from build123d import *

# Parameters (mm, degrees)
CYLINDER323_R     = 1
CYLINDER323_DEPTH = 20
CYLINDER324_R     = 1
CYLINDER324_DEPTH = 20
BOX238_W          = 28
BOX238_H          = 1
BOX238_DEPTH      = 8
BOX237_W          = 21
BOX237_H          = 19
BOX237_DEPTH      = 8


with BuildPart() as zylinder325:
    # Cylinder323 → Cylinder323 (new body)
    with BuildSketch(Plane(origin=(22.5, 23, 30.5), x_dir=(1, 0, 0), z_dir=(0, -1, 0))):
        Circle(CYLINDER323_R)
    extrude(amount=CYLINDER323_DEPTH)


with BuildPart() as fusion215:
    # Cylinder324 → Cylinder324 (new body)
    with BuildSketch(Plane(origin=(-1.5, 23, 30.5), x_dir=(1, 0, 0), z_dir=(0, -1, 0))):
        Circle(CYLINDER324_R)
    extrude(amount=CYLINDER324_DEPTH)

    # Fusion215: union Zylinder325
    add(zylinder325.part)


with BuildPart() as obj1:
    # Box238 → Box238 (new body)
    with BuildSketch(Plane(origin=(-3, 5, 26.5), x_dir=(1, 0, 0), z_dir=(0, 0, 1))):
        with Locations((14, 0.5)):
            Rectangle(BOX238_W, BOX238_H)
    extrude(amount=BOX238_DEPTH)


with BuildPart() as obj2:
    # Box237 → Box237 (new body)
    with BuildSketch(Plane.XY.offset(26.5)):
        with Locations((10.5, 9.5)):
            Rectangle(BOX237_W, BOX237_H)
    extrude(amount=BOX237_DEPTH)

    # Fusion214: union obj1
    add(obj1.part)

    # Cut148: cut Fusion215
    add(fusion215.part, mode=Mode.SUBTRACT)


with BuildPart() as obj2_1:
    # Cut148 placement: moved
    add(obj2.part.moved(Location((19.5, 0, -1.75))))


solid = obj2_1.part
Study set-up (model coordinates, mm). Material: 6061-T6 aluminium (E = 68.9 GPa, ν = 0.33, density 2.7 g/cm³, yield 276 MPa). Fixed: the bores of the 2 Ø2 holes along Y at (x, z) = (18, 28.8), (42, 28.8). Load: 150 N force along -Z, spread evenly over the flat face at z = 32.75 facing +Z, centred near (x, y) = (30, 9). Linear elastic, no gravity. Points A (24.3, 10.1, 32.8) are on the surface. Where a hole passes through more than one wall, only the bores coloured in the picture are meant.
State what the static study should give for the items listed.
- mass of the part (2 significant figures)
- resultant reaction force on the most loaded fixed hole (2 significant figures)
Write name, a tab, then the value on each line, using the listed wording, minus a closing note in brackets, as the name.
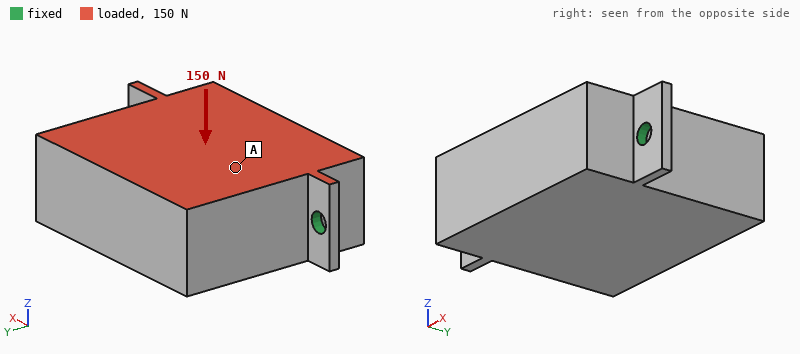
mass of the part	8.8 g
resultant reaction force on the most loaded fixed hole	75 N
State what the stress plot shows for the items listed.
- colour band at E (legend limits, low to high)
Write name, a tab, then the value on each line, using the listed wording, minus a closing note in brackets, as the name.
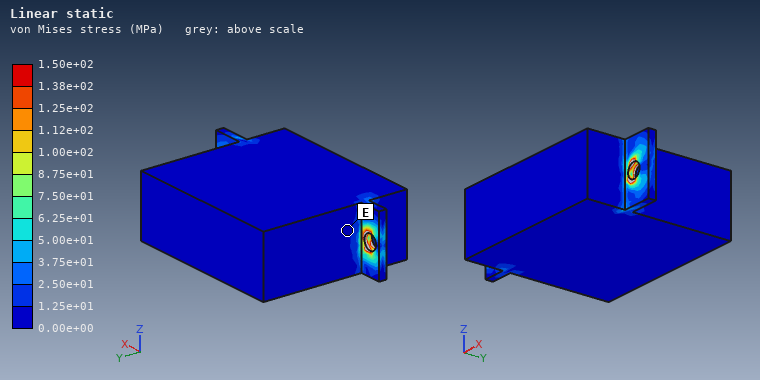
colour band at E	0.00e+00 to 1.25e+01 MPa
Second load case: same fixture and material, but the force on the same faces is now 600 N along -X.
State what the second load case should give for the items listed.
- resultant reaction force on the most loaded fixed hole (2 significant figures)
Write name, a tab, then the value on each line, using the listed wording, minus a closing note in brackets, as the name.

resultant reaction force on the most loaded fixed hole	340 N
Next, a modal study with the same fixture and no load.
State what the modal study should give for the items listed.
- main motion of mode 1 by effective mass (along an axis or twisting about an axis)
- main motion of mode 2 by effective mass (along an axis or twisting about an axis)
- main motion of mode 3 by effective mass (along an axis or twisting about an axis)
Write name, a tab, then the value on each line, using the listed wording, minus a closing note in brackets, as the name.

main motion of mode 1 by effective mass	along Z
main motion of mode 2 by effective mass	along Y
main motion of mode 3 by effective mass	along X
